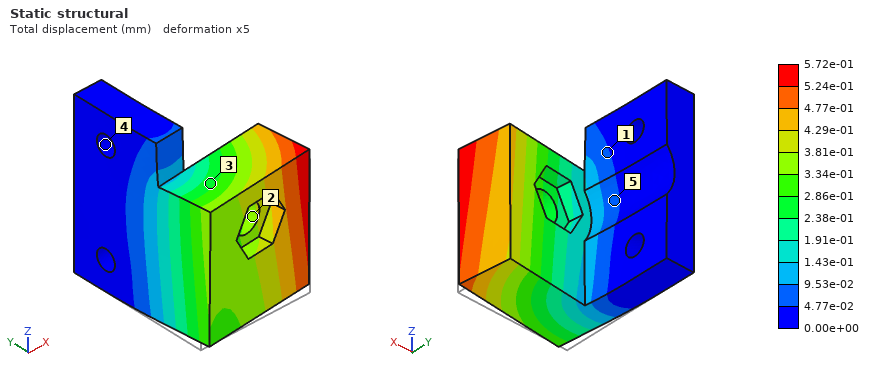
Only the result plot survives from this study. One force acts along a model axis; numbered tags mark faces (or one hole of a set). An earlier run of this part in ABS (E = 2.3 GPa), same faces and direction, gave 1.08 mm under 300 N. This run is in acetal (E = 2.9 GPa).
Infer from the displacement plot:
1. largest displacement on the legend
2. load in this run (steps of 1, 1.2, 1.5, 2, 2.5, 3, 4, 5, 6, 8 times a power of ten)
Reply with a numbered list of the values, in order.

1. 5.72e-01 mm
2. 200 N
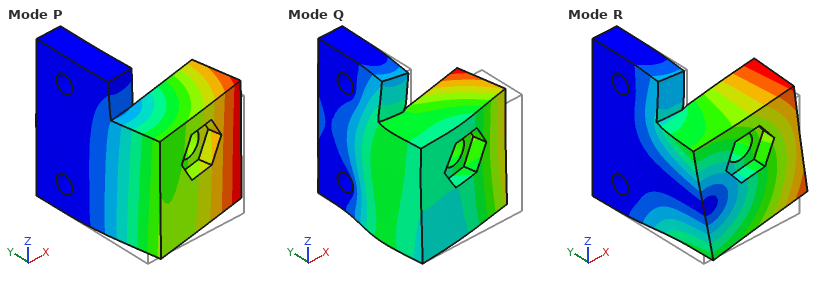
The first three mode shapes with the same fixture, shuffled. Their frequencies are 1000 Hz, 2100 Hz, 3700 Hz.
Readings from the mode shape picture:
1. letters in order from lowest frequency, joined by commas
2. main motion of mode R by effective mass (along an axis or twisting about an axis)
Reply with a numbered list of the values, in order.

1. P, R, Q
2. along Z
